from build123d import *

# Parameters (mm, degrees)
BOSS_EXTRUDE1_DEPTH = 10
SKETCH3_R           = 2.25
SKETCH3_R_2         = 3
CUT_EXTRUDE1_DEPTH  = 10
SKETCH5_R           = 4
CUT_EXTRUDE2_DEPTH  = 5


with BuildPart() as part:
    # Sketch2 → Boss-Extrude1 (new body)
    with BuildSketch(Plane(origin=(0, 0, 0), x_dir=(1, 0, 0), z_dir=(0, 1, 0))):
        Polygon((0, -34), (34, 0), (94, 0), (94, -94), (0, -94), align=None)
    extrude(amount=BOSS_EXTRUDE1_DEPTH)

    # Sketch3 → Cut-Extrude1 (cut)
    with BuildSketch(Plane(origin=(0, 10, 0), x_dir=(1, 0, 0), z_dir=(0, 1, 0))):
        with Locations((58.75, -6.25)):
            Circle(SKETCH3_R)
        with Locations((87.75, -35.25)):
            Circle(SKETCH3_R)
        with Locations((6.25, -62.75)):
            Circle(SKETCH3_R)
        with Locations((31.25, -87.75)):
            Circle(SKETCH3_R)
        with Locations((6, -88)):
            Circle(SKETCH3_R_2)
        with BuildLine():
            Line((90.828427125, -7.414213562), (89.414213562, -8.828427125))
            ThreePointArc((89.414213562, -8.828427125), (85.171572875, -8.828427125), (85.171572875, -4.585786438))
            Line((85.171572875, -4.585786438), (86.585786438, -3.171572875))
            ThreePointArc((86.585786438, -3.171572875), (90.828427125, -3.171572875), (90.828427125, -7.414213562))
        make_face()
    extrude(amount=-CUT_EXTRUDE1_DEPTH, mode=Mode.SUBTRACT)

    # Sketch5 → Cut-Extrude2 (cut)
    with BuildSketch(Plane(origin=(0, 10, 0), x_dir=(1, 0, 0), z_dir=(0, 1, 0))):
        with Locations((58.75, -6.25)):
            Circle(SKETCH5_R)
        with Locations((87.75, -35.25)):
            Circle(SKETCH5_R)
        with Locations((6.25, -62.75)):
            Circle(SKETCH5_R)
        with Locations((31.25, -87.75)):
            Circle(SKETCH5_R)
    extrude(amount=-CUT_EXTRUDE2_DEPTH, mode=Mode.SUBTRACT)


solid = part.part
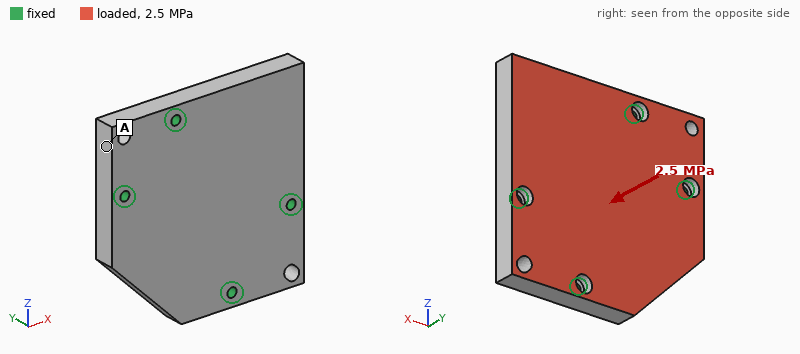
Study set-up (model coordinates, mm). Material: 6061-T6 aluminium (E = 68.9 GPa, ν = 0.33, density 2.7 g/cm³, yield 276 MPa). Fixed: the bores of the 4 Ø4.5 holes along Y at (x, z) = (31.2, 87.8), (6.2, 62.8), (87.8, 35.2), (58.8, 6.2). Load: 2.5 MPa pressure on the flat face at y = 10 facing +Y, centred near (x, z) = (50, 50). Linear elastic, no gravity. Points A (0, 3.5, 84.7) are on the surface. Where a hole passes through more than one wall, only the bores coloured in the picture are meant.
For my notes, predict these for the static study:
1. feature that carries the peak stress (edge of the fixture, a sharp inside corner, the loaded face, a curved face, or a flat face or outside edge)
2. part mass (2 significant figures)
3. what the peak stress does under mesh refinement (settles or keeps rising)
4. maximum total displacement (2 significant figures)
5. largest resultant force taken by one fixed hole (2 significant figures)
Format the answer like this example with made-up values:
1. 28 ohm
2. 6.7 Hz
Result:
1. edge of the fixture
2. 220 g
3. keeps rising
4. 0.37 mm
5. 7.3 kN
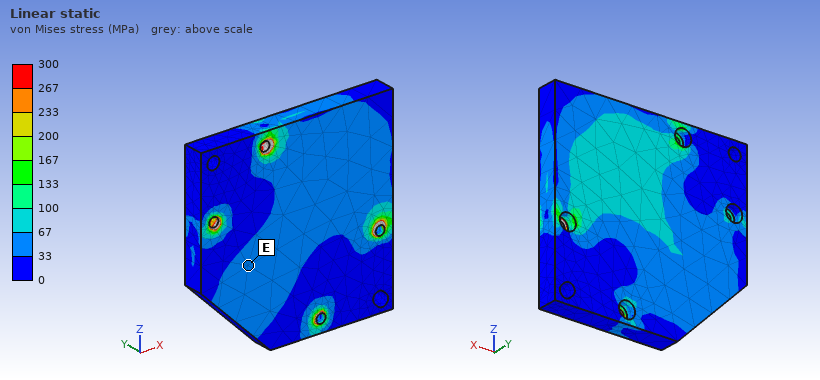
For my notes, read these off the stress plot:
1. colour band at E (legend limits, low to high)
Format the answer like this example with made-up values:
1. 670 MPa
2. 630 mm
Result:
1. 33 to 67 MPa
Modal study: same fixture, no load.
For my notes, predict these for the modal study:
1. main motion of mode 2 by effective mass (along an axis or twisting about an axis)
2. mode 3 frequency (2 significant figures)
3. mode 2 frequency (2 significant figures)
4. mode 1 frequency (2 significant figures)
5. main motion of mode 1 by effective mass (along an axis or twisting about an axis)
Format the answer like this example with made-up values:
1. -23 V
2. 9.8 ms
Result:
1. along Y
2. 8200 Hz
3. 5000 Hz
4. 3400 Hz
5. along Y
